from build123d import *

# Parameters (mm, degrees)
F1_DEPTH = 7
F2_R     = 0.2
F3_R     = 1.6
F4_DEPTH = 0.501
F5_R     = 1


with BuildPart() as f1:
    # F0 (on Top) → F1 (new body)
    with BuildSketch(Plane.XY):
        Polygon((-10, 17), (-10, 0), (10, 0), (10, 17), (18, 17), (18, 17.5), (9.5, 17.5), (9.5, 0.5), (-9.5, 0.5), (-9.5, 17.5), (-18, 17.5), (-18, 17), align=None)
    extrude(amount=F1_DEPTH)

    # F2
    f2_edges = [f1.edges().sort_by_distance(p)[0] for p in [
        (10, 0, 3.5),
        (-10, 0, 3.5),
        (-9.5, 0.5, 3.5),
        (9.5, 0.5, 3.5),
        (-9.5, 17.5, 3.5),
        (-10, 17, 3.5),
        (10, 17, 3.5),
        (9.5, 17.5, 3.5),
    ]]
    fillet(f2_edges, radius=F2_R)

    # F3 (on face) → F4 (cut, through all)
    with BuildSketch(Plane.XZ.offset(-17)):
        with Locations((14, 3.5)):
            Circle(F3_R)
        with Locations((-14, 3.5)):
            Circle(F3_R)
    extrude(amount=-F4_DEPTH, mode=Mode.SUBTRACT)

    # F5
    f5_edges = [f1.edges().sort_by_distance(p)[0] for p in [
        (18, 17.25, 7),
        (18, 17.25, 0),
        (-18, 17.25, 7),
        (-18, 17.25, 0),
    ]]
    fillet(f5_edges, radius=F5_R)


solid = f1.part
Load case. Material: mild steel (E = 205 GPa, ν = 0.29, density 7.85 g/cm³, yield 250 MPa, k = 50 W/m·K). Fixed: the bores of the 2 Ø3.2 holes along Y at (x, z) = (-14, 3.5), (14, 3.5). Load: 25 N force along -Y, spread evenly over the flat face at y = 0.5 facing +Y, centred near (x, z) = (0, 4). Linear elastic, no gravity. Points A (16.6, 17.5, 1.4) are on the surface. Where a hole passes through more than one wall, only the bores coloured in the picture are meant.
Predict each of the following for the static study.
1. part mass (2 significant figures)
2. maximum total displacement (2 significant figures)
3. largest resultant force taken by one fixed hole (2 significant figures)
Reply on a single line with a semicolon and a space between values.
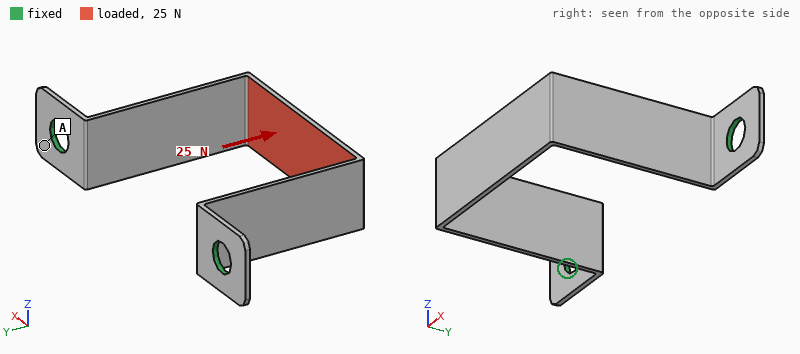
1.9 g; 74 µm; 13 N
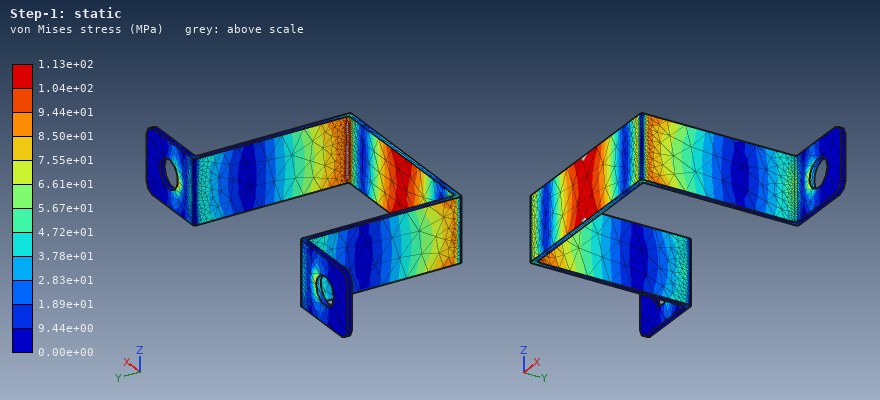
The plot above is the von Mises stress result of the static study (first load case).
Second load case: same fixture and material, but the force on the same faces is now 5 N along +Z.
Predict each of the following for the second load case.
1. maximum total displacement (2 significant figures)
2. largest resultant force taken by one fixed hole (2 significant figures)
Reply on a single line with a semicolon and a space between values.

54 µm; 2.5 N
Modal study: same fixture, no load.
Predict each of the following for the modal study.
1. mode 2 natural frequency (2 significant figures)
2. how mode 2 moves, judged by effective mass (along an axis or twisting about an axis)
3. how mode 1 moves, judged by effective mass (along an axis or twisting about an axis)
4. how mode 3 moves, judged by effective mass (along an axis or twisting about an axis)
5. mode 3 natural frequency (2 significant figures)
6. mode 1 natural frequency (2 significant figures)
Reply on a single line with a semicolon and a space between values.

1700 Hz; along Z; along X; twisting about Y; 2500 Hz; 1100 Hz
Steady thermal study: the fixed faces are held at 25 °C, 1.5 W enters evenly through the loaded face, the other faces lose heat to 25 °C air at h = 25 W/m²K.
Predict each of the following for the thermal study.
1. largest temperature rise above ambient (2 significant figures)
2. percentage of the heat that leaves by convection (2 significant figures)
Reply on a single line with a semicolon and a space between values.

73 K; 44 %
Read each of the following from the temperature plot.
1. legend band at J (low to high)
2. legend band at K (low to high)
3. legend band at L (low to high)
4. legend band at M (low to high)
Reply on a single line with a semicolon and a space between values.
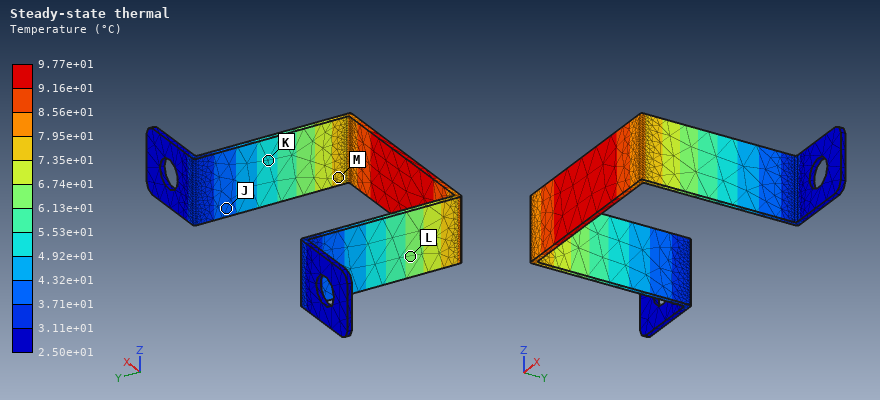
3.71e+01 to 4.32e+01 °C; 4.92e+01 to 5.53e+01 °C; 6.13e+01 to 6.74e+01 °C; 7.35e+01 to 7.95e+01 °C
